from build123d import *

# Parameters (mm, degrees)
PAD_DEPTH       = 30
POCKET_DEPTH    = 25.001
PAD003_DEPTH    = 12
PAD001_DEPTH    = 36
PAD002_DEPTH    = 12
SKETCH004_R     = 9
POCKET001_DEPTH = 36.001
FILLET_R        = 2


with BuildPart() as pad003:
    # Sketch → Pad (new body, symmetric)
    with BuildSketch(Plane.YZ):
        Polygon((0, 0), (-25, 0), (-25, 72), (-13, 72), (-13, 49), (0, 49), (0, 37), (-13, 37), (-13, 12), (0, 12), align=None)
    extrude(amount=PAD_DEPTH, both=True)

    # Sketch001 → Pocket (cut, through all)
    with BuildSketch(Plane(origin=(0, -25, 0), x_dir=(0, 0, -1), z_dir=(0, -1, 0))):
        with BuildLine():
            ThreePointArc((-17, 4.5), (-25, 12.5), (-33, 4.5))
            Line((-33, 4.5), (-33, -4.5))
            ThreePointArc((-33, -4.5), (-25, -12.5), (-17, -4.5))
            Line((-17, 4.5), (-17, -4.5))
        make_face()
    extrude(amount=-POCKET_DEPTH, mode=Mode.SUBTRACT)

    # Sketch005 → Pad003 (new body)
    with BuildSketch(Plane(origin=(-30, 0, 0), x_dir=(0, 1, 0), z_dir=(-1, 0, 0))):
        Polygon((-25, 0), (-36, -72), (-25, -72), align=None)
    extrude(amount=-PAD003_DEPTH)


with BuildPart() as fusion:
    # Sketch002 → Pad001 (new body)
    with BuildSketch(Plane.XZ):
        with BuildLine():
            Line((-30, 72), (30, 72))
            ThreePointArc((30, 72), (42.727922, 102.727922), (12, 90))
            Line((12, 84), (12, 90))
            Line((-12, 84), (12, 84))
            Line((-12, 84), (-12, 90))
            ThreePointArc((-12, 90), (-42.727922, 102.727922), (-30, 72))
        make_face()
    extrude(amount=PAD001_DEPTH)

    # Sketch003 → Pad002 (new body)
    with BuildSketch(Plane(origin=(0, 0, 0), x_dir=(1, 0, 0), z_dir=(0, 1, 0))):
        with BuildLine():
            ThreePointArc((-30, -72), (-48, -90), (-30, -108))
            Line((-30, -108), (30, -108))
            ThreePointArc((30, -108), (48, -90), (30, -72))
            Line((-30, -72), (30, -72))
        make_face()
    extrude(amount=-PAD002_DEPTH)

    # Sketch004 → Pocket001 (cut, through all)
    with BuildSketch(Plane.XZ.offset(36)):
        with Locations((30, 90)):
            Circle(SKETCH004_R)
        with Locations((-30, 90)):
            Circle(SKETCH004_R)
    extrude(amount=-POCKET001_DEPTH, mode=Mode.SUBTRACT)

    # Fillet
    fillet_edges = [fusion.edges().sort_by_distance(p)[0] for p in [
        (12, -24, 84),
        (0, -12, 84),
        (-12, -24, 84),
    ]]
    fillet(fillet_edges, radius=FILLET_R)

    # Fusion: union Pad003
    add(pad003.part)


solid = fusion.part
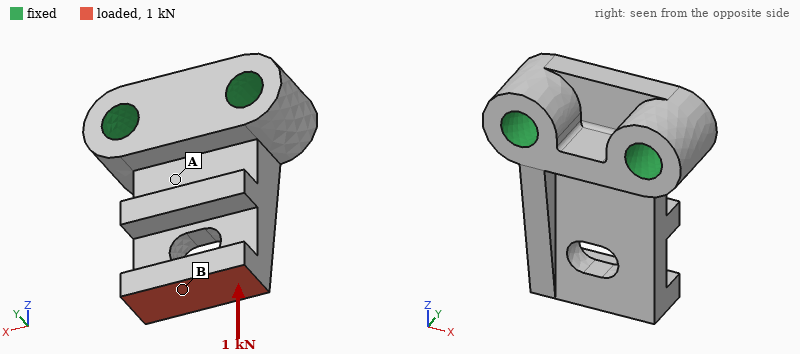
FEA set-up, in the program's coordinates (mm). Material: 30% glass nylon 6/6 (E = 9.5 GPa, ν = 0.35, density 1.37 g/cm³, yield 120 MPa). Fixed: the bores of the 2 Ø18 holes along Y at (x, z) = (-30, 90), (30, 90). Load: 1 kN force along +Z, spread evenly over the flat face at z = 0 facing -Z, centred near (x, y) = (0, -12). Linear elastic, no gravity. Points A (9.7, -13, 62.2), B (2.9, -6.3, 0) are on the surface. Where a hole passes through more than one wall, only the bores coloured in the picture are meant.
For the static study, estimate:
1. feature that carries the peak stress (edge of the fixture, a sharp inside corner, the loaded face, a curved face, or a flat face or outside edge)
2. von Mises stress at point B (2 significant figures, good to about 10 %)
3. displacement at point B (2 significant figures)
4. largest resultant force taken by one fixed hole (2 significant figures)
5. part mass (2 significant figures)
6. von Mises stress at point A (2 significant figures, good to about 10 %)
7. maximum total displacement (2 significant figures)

a curved face
1.4 MPa
0.18 mm
530 N
210 g
3.7 MPa
0.20 mm
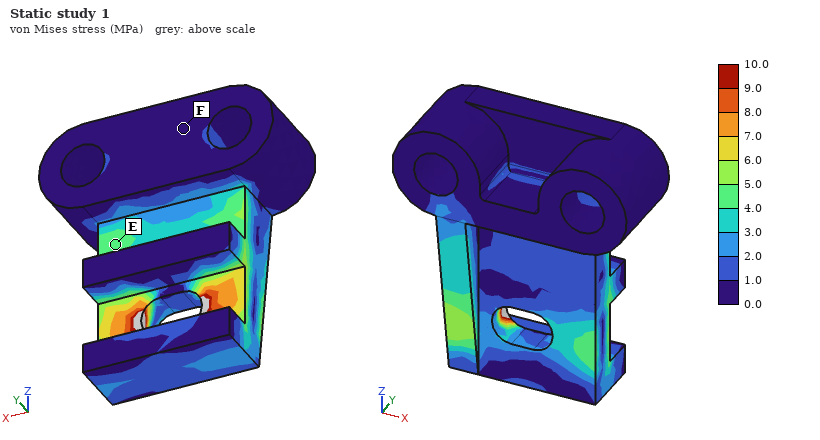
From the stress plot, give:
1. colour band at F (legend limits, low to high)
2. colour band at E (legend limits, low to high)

0.0 to 1.0 MPa
4.0 to 5.0 MPa
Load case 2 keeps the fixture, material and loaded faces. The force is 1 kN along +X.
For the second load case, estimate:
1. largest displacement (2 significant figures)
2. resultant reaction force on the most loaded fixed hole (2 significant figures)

0.20 mm
1.6 kN
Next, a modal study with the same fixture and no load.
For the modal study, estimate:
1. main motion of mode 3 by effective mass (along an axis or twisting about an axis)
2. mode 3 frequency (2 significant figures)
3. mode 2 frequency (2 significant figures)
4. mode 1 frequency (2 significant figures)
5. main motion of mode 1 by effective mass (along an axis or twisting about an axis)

along X
2600 Hz
2100 Hz
910 Hz
along Y
